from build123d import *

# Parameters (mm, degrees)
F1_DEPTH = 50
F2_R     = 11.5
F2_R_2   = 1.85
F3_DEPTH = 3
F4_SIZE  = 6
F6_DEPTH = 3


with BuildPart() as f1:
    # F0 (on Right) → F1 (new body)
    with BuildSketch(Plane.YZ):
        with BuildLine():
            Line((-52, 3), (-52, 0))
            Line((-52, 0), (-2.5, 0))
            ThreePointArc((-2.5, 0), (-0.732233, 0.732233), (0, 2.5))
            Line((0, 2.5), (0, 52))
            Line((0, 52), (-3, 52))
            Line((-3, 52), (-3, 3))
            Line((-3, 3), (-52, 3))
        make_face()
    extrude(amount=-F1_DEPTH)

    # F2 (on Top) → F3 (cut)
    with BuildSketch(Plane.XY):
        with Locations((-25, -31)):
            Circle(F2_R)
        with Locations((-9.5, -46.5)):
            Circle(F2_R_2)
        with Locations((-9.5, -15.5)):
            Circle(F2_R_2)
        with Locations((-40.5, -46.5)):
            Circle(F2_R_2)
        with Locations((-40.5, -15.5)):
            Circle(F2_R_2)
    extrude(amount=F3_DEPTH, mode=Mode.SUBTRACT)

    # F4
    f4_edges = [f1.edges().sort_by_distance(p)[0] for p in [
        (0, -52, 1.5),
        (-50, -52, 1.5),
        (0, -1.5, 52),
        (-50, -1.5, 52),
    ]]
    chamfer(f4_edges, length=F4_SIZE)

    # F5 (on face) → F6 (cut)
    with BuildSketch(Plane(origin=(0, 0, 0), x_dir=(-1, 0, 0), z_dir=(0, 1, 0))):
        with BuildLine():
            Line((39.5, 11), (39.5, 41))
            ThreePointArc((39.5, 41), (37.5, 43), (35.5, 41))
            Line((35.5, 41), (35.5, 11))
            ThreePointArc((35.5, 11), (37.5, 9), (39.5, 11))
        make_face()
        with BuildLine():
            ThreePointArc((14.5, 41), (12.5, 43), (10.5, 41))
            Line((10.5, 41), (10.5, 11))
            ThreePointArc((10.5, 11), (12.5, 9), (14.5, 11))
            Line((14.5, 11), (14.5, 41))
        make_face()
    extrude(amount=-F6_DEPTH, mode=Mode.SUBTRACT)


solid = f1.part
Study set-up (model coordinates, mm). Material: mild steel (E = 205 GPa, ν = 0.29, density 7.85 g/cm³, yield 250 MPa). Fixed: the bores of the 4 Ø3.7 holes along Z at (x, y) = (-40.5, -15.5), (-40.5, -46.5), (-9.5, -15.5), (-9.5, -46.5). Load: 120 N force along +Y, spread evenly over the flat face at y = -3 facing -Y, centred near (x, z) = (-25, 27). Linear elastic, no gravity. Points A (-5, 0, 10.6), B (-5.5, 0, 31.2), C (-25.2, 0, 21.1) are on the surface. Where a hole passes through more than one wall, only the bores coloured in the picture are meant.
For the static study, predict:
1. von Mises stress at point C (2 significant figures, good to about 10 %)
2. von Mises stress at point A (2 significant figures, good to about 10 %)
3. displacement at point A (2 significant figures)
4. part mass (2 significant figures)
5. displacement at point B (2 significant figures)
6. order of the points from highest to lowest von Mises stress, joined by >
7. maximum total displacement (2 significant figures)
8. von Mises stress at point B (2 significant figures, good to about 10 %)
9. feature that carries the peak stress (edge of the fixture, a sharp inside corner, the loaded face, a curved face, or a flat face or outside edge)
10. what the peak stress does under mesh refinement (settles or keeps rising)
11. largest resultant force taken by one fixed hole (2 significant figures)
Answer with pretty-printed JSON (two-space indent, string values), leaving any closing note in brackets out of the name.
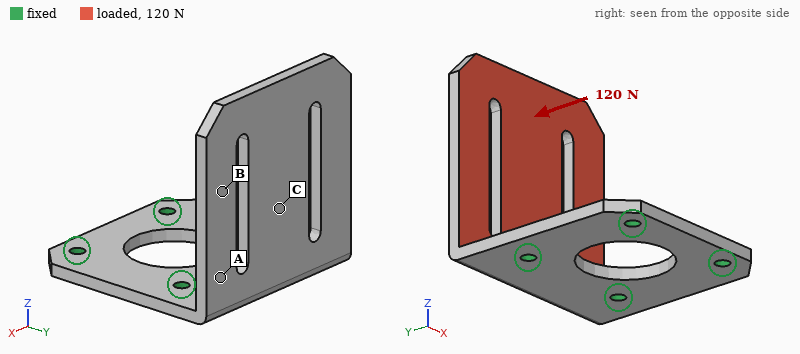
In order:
{
  "von Mises stress at point C": "18 MPa",
  "von Mises stress at point A": "30 MPa",
  "displacement at point A": "0.028 mm",
  "part mass": "100 g",
  "displacement at point B": "0.096 mm",
  "order of the points from highest to lowest von Mises stress, joined by >": "A > C > B",
  "maximum total displacement": "0.18 mm",
  "von Mises stress at point B": "8.9 MPa",
  "feature that carries the peak stress": "edge of the fixture",
  "what the peak stress does under mesh refinement": "keeps rising",
  "largest resultant force taken by one fixed hole": "60 N"
}
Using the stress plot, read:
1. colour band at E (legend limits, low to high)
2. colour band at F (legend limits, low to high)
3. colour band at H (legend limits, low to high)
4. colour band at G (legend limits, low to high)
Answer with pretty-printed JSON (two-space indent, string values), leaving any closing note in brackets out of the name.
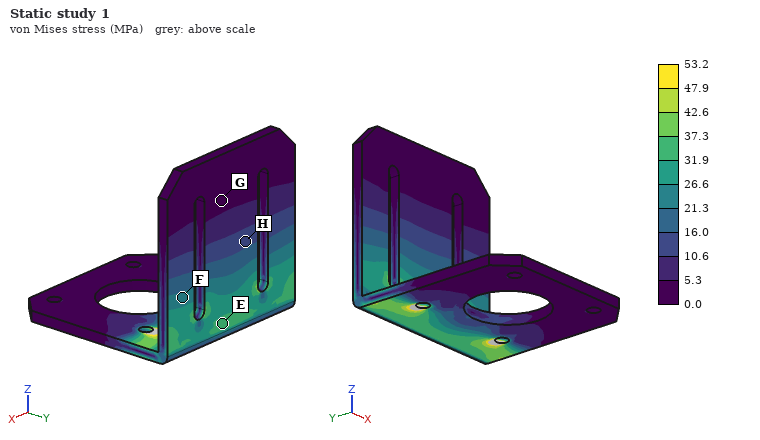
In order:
{
  "colour band at E": "31.9 to 37.3 MPa",
  "colour band at F": "21.3 to 26.6 MPa",
  "colour band at H": "10.6 to 16.0 MPa",
  "colour band at G": "0.0 to 5.3 MPa"
}
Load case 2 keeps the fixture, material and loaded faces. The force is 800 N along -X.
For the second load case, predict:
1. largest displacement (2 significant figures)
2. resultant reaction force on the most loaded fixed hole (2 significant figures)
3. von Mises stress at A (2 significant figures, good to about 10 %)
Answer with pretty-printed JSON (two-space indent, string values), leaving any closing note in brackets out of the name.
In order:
{
  "largest displacement": "0.13 mm",
  "resultant reaction force on the most loaded fixed hole": "780 N",
  "von Mises stress at A": "34 MPa"
}
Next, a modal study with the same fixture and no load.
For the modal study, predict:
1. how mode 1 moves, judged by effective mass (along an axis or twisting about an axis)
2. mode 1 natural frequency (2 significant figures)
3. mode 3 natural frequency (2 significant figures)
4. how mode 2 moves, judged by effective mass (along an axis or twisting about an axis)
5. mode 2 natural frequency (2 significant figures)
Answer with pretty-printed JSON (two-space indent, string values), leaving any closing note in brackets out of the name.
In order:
{
  "how mode 1 moves, judged by effective mass": "along Y",
  "mode 1 natural frequency": "700 Hz",
  "mode 3 natural frequency": "2600 Hz",
  "how mode 2 moves, judged by effective mass": "along X",
  "mode 2 natural frequency": "1800 Hz"
}
